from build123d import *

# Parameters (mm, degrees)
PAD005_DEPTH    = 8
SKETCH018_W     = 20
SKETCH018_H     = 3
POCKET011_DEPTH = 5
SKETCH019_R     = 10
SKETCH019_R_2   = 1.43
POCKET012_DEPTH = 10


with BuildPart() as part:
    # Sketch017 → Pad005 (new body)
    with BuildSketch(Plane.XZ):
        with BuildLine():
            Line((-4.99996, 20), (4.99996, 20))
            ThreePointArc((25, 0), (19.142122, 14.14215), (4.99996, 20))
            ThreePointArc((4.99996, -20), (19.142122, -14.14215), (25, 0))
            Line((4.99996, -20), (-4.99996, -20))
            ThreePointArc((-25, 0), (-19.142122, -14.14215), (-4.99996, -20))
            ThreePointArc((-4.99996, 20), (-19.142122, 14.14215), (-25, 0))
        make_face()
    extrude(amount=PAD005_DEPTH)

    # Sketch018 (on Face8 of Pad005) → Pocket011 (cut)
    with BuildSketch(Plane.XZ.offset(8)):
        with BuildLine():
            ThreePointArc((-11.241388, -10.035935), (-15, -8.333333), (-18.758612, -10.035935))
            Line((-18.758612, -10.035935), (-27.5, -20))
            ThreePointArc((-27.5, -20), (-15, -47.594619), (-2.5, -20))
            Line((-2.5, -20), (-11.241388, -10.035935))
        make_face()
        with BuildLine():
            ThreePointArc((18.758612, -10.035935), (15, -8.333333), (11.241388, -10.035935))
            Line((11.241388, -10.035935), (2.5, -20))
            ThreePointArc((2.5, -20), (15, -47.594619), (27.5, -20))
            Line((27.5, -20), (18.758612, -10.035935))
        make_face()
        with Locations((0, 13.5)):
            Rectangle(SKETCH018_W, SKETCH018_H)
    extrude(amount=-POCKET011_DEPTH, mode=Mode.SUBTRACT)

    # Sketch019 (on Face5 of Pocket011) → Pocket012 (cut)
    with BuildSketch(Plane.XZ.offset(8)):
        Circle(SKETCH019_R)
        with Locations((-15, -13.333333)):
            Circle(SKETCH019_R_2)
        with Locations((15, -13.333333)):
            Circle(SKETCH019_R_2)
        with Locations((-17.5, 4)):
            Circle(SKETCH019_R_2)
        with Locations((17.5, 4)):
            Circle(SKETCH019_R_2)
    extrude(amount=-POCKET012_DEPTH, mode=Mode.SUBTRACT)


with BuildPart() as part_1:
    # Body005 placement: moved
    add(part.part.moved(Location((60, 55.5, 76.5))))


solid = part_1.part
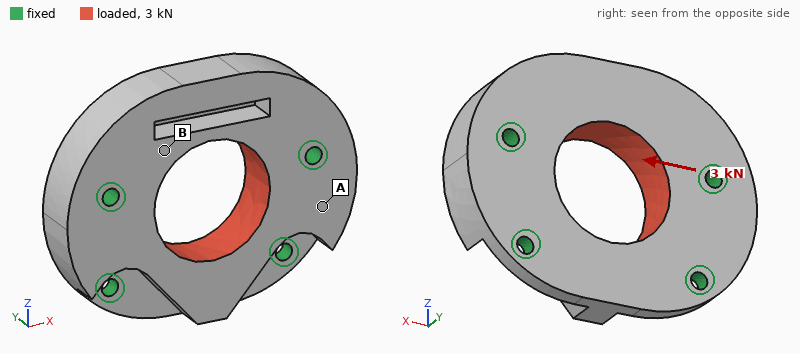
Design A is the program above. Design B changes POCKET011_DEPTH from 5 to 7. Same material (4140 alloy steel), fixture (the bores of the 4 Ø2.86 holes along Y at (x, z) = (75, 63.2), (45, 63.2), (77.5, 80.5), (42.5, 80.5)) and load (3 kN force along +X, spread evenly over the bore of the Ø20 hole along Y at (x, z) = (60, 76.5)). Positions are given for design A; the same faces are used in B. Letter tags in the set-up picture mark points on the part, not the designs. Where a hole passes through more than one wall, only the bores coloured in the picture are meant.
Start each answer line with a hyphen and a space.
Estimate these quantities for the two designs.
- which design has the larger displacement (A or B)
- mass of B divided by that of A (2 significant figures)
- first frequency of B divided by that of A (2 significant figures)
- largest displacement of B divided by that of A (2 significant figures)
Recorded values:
- B
- 0.94
- 0.78
- 1.7
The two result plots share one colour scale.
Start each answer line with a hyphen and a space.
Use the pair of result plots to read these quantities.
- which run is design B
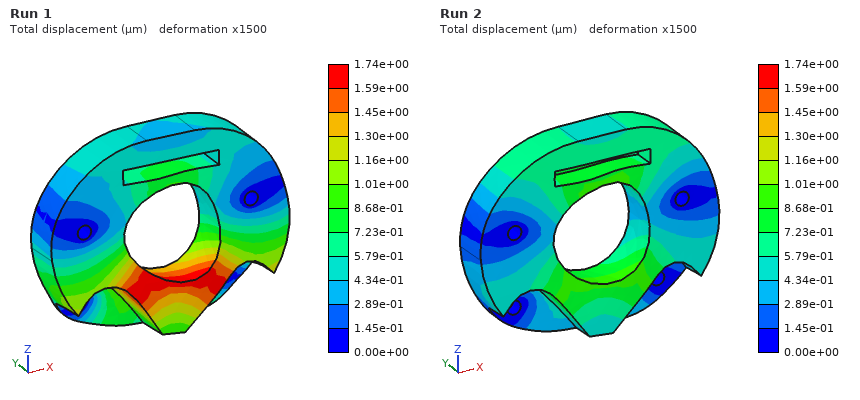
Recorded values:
- Run 1
